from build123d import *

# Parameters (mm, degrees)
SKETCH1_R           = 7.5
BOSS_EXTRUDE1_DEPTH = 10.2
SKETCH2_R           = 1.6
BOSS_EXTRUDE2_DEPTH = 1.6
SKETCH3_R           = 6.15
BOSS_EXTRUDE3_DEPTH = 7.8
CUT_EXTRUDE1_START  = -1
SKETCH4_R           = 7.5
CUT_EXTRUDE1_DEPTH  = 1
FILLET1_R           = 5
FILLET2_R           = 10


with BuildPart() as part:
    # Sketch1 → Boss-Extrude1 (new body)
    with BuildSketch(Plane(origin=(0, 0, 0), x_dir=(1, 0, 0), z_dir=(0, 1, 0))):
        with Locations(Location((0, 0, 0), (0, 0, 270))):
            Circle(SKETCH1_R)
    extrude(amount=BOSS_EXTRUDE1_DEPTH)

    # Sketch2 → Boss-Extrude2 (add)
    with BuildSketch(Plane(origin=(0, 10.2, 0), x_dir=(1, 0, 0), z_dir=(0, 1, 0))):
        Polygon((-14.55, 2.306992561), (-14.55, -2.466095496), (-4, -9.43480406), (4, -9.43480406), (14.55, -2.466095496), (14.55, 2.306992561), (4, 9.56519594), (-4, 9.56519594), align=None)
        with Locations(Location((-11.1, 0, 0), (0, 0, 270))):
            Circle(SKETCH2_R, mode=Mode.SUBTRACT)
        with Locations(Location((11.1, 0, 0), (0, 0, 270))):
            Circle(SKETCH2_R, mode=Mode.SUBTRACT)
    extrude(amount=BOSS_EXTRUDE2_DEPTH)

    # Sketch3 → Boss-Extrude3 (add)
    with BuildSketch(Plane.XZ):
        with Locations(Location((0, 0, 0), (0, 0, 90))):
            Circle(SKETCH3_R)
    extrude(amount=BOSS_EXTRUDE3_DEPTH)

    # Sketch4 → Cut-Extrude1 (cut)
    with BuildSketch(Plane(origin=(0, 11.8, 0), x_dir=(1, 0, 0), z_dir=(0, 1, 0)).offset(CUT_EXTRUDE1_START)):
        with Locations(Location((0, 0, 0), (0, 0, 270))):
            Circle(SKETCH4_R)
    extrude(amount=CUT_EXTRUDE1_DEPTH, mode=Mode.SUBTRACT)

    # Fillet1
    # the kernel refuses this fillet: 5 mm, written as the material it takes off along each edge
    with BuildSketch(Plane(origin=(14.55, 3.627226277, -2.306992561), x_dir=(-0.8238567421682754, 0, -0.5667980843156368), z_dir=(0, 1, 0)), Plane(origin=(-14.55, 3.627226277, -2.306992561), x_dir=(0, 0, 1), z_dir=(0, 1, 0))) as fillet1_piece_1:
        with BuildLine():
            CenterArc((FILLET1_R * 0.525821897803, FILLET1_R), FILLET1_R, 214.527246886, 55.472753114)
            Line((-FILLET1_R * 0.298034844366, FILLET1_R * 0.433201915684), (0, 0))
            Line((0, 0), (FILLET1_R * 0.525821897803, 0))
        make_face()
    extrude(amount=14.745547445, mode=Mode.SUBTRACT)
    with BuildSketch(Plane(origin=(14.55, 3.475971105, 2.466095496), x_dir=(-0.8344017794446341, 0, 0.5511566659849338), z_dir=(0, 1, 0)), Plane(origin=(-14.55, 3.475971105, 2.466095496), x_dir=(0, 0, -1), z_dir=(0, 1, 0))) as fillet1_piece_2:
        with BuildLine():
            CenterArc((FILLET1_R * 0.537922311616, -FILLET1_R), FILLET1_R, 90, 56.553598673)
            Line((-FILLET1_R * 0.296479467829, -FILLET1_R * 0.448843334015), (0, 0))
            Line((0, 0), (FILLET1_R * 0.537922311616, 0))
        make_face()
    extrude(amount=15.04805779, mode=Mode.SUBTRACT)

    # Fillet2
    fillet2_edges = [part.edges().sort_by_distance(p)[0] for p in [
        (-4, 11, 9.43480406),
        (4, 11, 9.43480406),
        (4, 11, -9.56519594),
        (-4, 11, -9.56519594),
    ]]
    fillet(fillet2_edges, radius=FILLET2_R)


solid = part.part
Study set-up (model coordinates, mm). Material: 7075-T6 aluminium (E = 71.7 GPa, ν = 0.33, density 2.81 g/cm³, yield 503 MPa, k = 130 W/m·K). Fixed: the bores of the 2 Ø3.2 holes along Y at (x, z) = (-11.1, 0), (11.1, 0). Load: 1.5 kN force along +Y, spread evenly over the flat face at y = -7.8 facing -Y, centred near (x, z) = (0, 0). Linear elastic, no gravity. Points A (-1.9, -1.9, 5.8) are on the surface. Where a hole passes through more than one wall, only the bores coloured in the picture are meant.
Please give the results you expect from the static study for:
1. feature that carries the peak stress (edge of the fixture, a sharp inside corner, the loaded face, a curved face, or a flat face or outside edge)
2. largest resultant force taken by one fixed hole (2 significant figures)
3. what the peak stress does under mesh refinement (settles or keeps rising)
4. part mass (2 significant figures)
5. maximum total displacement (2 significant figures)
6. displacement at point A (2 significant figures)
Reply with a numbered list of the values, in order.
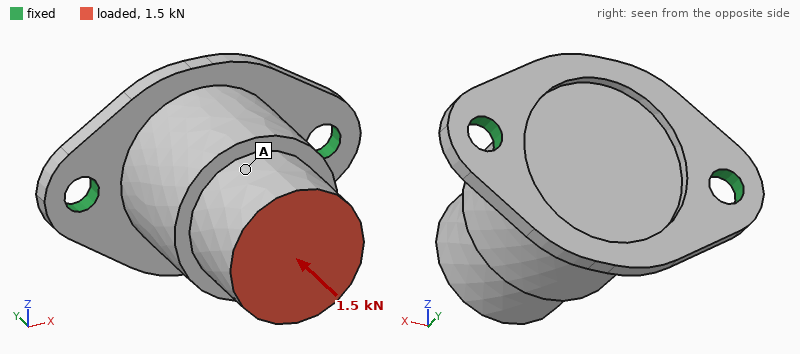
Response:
1. edge of the fixture
2. 960 N
3. keeps rising
4. 8.9 g
5. 29 µm
6. 28 µm
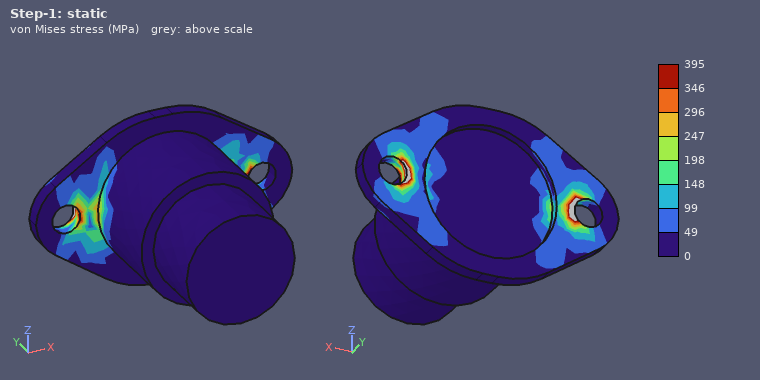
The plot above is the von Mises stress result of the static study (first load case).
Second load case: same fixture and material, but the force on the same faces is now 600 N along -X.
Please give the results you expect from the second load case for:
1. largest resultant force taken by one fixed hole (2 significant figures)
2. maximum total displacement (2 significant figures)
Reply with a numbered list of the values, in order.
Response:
1. 740 N
2. 69 µm
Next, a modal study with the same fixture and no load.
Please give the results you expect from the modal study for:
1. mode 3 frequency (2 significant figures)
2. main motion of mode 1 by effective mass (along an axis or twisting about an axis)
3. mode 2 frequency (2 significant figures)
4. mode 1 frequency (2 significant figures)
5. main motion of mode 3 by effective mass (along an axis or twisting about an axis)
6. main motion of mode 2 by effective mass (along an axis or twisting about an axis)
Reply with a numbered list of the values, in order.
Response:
1. 13 kHz
2. along Z
3. 9900 Hz
4. 2800 Hz
5. along Y
6. along X
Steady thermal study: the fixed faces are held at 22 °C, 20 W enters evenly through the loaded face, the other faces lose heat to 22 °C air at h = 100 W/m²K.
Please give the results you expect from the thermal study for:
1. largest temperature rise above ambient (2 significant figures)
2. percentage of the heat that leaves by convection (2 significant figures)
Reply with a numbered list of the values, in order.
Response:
1. 40 K
2. 18 %
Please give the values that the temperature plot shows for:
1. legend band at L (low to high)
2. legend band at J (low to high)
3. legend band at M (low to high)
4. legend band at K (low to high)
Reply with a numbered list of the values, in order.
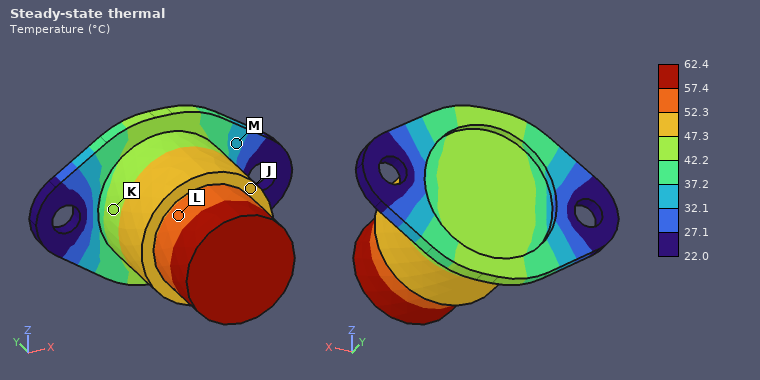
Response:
1. 52.3 to 57.4 °C
2. 47.3 to 52.3 °C
3. 32.1 to 37.2 °C
4. 42.2 to 47.3 °C
